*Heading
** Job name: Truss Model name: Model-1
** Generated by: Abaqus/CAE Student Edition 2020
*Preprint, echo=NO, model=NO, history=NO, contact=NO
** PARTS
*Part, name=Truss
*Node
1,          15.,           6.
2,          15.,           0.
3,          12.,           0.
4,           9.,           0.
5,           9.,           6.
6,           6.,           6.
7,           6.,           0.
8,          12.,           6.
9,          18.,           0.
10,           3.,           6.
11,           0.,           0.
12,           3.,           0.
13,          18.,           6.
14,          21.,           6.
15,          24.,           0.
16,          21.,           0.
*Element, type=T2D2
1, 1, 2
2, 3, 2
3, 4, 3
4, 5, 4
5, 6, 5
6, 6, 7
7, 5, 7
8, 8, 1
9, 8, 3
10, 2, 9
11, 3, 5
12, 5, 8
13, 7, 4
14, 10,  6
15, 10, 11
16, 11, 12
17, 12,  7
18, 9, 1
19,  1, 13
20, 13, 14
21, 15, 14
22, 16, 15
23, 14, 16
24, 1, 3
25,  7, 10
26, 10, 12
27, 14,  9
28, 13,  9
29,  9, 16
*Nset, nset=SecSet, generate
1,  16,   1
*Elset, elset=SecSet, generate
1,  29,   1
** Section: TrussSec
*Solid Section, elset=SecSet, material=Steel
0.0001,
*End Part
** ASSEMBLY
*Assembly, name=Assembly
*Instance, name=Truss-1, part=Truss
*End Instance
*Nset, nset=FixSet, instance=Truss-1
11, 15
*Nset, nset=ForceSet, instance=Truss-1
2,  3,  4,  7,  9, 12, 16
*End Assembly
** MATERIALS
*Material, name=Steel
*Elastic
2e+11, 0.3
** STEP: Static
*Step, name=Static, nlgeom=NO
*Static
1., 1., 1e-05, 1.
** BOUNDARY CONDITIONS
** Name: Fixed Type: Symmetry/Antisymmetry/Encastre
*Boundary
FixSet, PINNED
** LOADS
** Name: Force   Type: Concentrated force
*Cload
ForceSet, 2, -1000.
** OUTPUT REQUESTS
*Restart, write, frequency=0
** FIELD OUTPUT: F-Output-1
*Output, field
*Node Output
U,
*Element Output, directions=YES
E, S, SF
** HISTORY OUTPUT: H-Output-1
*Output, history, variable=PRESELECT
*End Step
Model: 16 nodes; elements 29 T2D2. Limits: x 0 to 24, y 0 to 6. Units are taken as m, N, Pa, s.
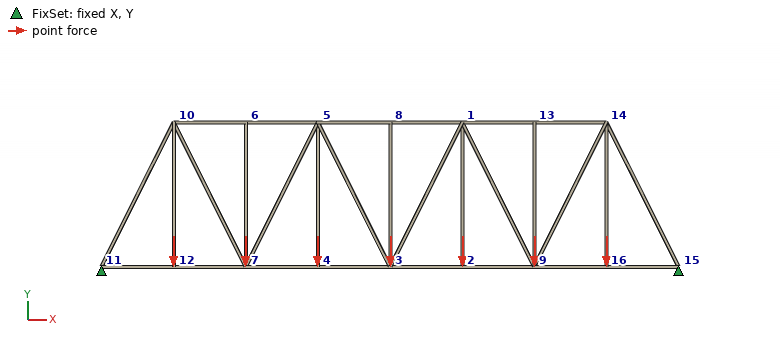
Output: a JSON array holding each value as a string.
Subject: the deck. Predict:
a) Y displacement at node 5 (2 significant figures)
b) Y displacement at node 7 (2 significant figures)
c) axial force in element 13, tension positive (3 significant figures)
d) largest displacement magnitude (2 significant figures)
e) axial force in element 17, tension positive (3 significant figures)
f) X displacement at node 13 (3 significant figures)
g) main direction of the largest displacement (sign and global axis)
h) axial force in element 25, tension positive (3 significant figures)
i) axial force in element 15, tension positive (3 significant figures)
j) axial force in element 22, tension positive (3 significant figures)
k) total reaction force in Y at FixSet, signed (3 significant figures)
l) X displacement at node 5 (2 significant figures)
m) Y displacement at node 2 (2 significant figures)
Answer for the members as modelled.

["-0.0052 m", "-0.0042 m", "1000 N", "0.0058 m", "-1000 N", "-0.00105 m", "-Y", "2800 N", "-3910 N", "-1000 N", "7000 N", "6.0e-04 m", "-0.0055 m"]
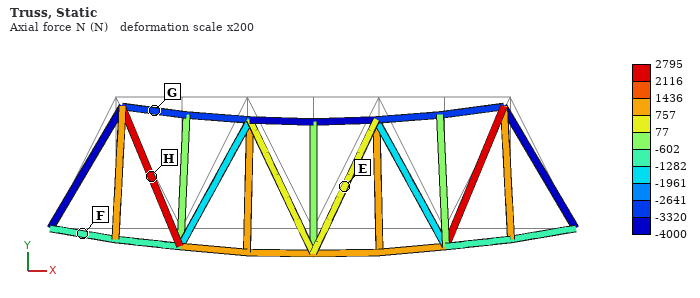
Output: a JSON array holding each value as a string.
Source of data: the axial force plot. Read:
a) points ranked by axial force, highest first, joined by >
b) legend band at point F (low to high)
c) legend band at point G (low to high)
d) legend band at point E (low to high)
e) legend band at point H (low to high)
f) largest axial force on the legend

["H > E > F > G", "-1282 to -602 N", "-3320 to -2641 N", "77 to 757 N", "2116 to 2795 N", "2795 N"]
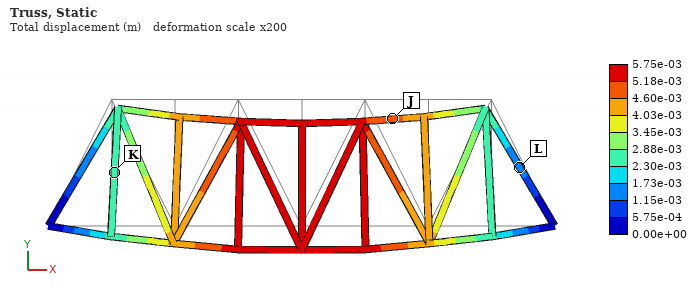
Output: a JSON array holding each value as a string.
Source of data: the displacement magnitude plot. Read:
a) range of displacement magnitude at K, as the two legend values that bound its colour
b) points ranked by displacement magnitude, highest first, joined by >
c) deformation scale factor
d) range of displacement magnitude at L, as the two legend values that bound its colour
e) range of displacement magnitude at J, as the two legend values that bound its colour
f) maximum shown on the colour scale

["2.30e-03 to 2.88e-03 m", "J > K > L", "200", "1.15e-03 to 1.73e-03 m", "4.60e-03 to 5.18e-03 m", "5.75e-03 m"]
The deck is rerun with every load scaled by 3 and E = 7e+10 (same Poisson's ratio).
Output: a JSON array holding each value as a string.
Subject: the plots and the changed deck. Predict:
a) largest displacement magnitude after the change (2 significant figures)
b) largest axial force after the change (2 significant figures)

["0.049 m", "8400 N"]
